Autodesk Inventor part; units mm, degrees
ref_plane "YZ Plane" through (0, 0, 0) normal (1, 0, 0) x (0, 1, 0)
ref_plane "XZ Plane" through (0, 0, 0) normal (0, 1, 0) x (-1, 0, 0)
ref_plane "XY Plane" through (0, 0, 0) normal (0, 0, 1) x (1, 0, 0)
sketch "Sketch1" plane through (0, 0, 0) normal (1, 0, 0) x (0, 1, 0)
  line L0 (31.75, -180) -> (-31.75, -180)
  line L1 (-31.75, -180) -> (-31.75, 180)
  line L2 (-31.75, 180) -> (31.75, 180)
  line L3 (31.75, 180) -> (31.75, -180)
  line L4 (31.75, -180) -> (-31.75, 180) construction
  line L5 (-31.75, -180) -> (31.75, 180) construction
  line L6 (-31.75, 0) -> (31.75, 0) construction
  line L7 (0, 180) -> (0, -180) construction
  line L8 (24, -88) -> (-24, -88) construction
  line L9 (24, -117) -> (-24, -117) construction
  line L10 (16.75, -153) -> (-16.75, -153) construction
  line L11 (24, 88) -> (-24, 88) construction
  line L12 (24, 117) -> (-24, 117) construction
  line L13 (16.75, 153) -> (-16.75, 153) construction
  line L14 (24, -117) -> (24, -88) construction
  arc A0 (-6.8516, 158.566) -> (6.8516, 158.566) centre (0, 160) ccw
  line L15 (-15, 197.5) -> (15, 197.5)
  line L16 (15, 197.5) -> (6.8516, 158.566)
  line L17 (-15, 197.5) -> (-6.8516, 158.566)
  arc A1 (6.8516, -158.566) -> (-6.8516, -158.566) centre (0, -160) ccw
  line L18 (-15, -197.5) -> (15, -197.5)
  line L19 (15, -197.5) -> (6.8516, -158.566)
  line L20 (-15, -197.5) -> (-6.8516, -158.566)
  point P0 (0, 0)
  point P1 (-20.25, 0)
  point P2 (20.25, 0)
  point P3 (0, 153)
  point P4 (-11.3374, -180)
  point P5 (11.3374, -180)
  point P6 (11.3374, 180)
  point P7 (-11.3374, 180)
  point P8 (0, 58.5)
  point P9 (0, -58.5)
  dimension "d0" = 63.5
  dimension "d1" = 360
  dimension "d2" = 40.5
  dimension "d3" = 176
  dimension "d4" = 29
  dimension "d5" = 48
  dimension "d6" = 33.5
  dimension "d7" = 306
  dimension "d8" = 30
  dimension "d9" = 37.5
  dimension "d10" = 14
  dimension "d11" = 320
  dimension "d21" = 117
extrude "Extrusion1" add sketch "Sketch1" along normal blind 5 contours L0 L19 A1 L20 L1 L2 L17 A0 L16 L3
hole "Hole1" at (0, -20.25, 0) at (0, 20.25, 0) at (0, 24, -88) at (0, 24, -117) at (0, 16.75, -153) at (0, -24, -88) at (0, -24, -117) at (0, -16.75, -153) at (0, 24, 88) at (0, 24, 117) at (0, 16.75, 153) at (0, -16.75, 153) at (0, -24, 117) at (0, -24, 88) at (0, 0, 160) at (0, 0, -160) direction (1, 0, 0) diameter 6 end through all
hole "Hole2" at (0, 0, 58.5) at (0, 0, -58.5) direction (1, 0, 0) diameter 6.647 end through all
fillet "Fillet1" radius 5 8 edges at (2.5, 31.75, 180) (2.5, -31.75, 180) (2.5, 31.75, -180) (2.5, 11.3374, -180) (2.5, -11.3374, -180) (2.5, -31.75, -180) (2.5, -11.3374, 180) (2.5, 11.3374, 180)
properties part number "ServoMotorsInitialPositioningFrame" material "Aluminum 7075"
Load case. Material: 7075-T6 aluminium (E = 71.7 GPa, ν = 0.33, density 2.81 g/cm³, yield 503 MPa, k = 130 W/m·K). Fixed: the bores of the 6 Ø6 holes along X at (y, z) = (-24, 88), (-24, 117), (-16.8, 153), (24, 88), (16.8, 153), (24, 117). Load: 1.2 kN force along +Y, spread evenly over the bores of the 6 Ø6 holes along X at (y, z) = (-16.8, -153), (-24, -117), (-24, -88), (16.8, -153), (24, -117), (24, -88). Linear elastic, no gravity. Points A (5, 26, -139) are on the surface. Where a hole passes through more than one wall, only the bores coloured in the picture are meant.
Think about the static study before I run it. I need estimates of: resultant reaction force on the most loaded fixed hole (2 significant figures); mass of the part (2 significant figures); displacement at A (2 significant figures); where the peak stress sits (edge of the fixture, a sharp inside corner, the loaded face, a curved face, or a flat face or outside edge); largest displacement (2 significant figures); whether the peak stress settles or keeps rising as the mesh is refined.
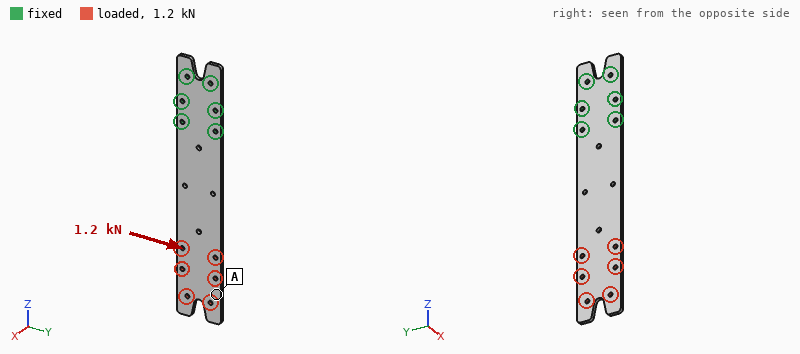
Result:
4.7 kN
300 g
0.59 mm
edge of the fixture
0.74 mm
keeps rising
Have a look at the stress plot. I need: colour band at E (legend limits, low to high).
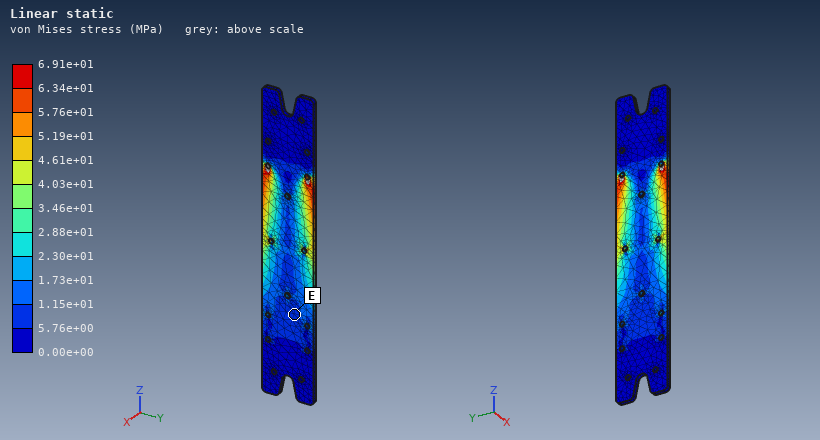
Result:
5.76e+00 to 1.15e+01 MPa
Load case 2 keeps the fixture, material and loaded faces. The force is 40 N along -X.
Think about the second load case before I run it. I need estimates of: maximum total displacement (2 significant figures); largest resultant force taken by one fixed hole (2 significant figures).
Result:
3.7 mm
66 N
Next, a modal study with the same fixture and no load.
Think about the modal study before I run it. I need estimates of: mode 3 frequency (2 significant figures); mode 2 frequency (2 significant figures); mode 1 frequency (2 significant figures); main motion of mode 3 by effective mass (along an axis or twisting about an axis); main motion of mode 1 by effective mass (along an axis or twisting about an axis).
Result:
470 Hz
370 Hz
60 Hz
twisting about Z
along X
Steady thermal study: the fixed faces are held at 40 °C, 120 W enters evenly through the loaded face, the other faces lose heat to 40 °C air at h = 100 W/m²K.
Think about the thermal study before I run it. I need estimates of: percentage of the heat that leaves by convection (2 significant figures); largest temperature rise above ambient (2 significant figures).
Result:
97 %
75 K
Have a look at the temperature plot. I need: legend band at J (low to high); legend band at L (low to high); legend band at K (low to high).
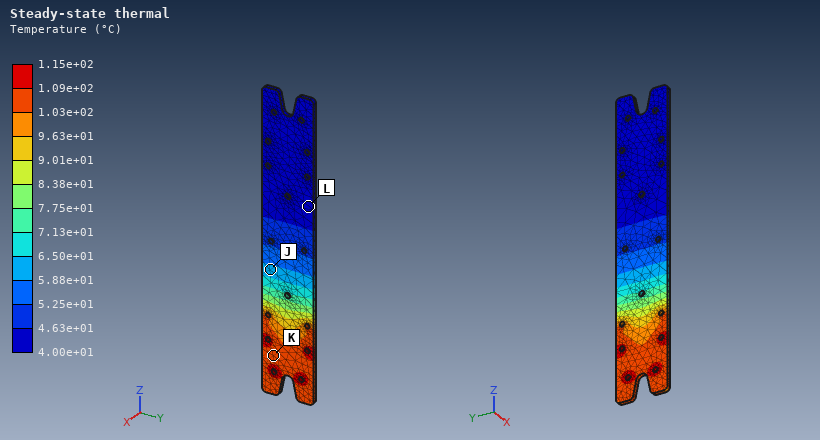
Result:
5.88e+01 to 6.50e+01 °C
4.00e+01 to 4.63e+01 °C
1.03e+02 to 1.09e+02 °C
